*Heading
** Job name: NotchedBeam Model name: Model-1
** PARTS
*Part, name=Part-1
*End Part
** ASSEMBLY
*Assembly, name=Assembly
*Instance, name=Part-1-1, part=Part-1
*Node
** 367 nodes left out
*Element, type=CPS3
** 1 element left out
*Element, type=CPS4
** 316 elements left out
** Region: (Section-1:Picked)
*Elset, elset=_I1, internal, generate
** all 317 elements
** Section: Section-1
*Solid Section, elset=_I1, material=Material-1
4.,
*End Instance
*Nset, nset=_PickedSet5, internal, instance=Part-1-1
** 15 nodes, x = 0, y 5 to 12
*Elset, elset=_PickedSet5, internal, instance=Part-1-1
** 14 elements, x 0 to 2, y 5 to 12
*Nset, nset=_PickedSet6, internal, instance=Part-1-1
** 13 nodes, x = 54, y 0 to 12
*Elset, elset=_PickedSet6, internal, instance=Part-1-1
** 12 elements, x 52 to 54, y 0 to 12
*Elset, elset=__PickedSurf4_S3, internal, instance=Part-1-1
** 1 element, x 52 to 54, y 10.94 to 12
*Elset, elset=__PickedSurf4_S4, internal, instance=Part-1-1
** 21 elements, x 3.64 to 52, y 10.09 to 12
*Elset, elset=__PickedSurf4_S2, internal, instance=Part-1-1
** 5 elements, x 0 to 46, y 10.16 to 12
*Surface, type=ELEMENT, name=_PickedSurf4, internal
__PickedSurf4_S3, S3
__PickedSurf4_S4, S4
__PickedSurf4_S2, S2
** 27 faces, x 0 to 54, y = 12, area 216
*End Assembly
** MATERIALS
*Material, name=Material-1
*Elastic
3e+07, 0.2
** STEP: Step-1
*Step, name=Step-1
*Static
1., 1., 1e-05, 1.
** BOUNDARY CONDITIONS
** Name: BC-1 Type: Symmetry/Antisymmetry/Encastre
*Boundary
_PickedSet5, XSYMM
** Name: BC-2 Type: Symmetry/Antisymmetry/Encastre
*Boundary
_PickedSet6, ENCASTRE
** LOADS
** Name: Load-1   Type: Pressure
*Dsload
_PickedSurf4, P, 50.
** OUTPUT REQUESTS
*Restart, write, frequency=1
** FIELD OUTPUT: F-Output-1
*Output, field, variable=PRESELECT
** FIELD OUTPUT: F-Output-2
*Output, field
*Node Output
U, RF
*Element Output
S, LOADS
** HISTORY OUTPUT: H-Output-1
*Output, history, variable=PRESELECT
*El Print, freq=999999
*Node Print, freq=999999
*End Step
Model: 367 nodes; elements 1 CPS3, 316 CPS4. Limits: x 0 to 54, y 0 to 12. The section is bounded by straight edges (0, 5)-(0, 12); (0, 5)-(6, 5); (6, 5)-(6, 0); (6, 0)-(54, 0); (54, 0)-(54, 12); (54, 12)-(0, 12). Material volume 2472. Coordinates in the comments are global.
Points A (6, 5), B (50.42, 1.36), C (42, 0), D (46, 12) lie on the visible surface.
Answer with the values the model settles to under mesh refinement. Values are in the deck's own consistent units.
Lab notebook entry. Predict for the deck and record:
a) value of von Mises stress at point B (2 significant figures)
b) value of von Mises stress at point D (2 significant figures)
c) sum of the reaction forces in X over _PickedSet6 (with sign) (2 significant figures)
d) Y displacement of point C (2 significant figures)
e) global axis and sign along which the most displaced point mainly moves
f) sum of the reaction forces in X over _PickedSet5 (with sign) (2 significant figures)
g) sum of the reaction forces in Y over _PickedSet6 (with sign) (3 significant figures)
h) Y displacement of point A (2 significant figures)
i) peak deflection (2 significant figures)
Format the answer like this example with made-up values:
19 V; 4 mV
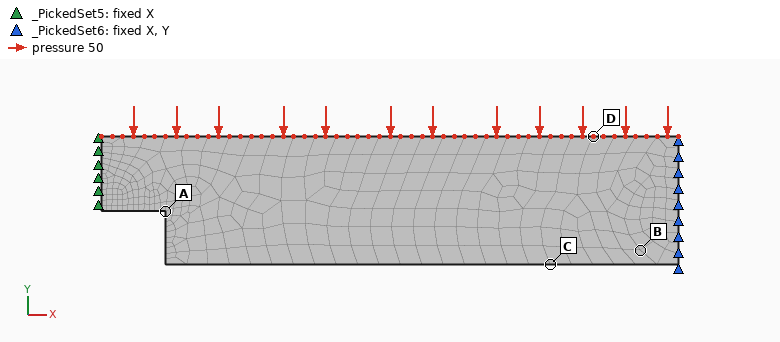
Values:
1700; 1300; -7500; -1.0e-03; -Y; 7500; 10800; -0.0065; 0.0067
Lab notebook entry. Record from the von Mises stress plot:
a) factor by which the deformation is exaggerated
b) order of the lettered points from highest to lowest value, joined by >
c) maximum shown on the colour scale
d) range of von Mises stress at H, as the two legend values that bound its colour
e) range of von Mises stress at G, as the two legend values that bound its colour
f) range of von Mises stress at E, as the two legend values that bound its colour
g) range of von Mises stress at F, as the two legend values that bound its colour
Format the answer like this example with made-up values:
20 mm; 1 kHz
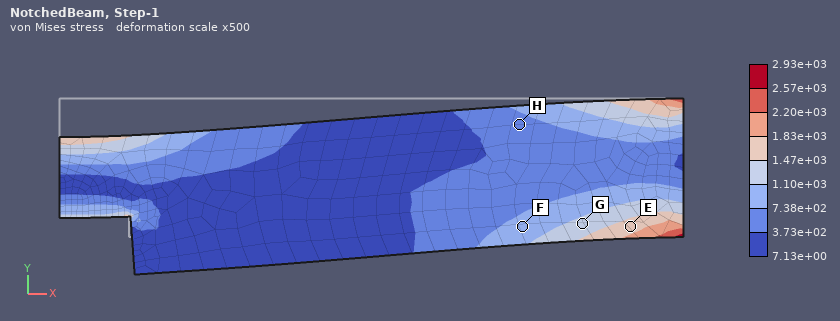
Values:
500; E > G > F > H; 2.93e+03; 3.73e+02 to 7.38e+02; 1.10e+03 to 1.47e+03; 1.47e+03 to 1.83e+03; 7.38e+02 to 1.10e+03
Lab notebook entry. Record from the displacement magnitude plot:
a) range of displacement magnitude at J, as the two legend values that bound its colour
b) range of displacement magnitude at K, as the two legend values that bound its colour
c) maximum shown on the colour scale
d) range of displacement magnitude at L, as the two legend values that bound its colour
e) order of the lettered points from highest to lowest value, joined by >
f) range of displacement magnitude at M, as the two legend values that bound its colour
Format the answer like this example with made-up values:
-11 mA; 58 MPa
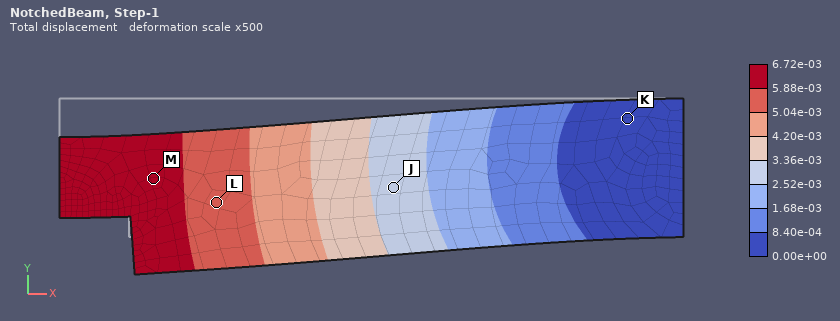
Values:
2.52e-03 to 3.36e-03; 0.00e+00 to 8.40e-04; 6.72e-03; 5.04e-03 to 5.88e-03; M > L > J > K; 5.88e-03 to 6.72e-03
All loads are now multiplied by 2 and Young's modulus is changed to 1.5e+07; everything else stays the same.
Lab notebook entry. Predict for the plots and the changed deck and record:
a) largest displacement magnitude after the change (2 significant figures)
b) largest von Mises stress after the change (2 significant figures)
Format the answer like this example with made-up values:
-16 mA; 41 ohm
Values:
0.027; 5900
